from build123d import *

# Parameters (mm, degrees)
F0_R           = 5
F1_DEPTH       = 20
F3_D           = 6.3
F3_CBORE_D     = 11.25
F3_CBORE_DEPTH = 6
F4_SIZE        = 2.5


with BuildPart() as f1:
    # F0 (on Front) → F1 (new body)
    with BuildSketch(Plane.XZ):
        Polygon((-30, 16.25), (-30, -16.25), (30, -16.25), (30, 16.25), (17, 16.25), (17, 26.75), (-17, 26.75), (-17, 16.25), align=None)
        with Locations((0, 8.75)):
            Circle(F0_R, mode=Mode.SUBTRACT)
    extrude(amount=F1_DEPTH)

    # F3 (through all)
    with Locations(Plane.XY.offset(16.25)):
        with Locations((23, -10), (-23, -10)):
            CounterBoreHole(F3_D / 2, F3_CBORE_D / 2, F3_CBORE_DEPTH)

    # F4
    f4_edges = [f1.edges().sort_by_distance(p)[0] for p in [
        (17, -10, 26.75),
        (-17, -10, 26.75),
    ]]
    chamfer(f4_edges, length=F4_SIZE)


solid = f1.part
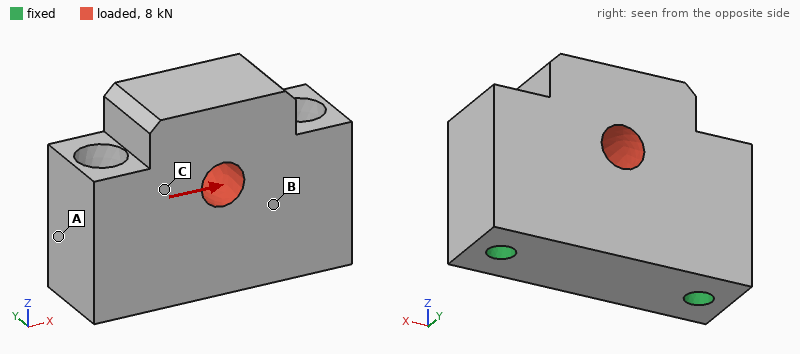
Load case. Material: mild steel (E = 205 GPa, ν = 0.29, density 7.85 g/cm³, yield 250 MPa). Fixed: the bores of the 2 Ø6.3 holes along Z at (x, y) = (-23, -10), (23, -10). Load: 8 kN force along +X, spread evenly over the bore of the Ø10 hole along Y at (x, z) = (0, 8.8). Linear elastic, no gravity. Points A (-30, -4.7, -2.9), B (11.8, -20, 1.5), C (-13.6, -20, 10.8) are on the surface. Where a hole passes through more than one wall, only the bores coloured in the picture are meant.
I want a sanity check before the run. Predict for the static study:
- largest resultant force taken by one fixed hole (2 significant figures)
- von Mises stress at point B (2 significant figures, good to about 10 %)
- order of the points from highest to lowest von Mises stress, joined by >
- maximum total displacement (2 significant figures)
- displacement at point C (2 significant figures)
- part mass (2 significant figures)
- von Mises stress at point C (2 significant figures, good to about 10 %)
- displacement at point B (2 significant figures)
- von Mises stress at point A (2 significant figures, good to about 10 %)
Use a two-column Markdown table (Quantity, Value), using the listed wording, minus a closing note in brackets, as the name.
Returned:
| Quantity | Value |
|---|---|
| largest resultant force taken by one fixed hole | 4.2 kN |
| von Mises stress at point B | 7.6 MPa |
| order of the points from highest to lowest von Mises stress, joined by > | C > B > A |
| maximum total displacement | 1.8 µm |
| displacement at point C | 0.94 µm |
| part mass | 330 g |
| von Mises stress at point C | 12 MPa |
| displacement at point B | 0.52 µm |
| von Mises stress at point A | 3.3 MPa |
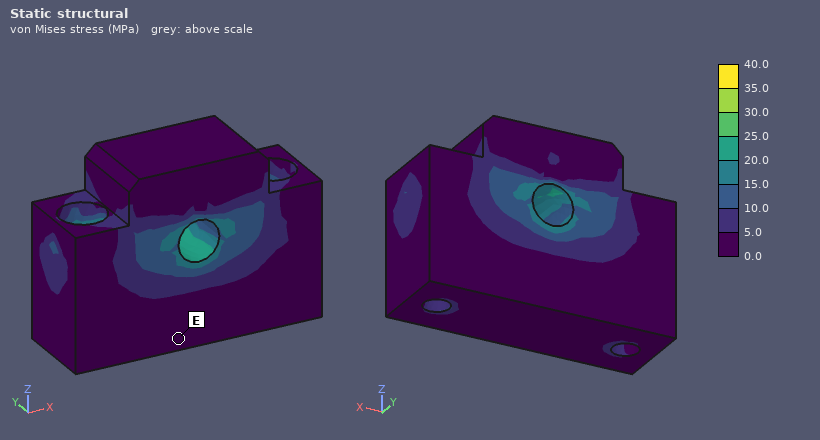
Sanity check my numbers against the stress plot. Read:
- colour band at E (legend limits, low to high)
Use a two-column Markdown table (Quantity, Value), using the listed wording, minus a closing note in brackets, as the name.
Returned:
| Quantity | Value |
|---|---|
| colour band at E | 0.0 to 5.0 MPa |
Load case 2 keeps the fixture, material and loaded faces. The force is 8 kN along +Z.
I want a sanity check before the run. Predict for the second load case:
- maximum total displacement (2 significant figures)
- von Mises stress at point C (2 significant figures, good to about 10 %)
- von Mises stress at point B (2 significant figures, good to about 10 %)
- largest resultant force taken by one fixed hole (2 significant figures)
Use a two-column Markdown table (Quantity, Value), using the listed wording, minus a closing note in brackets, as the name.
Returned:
| Quantity | Value |
|---|---|
| maximum total displacement | 2.3 µm |
| von Mises stress at point C | 7.6 MPa |
| von Mises stress at point B | 11 MPa |
| largest resultant force taken by one fixed hole | 4.2 kN |
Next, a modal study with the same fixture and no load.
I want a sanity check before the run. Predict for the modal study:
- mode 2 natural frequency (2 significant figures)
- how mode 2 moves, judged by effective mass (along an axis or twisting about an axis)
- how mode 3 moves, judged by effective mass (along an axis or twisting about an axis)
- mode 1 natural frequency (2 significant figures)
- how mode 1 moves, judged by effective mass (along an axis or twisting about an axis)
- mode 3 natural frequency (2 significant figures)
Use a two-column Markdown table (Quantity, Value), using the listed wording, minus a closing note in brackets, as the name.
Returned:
| Quantity | Value |
|---|---|
| mode 2 natural frequency | 25 kHz |
| how mode 2 moves, judged by effective mass | along Y |
| how mode 3 moves, judged by effective mass | along Z |
| mode 1 natural frequency | 14 kHz |
| how mode 1 moves, judged by effective mass | along Y |
| mode 3 natural frequency | 27 kHz |
